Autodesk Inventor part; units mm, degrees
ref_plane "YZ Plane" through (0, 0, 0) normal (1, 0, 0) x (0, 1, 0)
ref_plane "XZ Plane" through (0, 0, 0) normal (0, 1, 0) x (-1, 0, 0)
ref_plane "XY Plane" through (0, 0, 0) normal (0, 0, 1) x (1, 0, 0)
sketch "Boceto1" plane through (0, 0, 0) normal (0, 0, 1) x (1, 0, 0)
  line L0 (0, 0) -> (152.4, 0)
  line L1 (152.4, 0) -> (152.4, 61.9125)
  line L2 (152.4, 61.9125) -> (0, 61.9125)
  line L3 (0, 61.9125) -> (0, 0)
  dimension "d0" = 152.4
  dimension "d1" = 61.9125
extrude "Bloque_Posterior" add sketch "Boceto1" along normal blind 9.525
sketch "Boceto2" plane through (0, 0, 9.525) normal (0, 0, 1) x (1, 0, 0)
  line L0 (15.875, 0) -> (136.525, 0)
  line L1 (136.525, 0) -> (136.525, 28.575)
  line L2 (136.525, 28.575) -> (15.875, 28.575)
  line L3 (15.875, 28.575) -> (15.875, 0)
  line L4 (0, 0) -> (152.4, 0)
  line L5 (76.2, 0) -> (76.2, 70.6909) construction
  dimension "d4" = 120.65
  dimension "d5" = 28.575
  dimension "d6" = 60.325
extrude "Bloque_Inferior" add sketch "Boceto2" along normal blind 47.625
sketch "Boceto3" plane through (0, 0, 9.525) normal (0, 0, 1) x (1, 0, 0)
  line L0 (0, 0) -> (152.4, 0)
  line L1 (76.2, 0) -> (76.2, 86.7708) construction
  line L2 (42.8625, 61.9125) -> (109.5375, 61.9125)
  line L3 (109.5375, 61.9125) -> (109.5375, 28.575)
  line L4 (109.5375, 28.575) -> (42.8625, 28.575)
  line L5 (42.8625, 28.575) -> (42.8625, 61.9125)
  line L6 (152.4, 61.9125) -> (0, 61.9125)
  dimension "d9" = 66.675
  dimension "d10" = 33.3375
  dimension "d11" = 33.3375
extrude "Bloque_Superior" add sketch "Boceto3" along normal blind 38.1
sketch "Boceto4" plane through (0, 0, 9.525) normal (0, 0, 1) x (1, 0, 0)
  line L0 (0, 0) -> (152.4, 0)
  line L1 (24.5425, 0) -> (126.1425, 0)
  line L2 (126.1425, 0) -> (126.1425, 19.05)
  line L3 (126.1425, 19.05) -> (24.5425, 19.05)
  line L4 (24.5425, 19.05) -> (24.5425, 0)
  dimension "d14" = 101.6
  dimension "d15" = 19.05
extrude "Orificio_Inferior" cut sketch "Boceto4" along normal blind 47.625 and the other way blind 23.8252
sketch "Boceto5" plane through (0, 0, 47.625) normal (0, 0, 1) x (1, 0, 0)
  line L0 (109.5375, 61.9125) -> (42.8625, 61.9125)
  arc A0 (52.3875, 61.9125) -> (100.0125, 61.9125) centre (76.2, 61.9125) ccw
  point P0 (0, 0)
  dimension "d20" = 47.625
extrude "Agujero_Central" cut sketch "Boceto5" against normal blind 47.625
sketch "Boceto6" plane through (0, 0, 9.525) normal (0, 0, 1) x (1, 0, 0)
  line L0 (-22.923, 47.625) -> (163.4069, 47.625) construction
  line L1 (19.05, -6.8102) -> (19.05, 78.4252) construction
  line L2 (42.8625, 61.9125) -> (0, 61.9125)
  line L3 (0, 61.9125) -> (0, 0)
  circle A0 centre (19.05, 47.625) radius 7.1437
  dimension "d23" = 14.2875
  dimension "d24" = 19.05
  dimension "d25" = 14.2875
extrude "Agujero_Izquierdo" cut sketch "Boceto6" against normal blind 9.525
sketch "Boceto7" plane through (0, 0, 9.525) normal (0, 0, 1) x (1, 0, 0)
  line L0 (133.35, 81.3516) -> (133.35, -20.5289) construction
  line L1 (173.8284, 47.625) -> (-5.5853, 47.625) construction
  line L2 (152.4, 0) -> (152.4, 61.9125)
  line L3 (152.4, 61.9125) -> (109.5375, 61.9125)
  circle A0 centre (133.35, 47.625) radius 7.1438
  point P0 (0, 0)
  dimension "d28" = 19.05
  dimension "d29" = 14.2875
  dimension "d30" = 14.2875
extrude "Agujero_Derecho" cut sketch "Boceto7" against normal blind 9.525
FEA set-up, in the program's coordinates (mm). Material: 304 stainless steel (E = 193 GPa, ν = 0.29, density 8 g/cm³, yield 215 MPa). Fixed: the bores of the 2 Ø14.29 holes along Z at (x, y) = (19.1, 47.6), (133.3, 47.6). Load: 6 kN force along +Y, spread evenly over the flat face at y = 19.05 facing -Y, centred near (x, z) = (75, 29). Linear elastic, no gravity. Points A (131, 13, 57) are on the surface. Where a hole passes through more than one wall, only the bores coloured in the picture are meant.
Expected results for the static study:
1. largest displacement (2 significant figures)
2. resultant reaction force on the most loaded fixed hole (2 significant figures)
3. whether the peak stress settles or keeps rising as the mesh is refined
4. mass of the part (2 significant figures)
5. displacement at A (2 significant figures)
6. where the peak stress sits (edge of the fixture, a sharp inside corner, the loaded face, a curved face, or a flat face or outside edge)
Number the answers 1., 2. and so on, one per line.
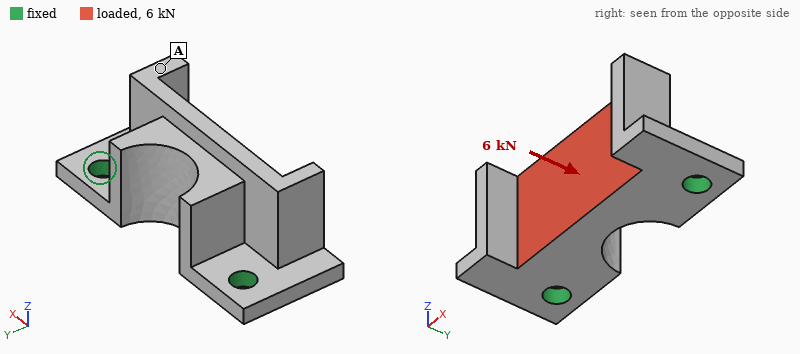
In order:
1. 74 µm
2. 3.6 kN
3. keeps rising
4. 1.5 kg
5. 65 µm
6. edge of the fixture
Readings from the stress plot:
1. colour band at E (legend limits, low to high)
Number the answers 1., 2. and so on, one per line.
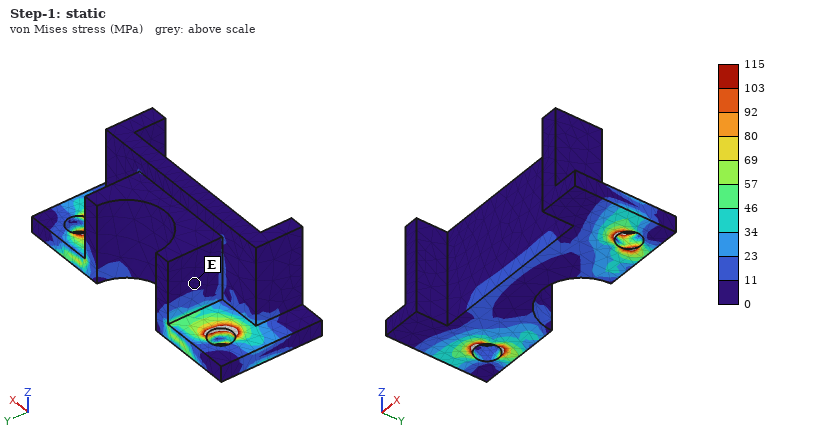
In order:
1. 0 to 11 MPa
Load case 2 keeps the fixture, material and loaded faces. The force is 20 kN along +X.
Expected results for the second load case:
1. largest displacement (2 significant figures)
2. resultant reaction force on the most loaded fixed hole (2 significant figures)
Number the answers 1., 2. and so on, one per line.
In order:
1. 21 µm
2. 12 kN
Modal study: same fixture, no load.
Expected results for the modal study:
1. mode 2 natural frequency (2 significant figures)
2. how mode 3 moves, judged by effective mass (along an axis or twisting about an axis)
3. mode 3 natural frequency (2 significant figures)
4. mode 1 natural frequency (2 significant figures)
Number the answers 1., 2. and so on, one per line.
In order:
1. 3400 Hz
2. along Z
3. 4600 Hz
4. 1600 Hz
